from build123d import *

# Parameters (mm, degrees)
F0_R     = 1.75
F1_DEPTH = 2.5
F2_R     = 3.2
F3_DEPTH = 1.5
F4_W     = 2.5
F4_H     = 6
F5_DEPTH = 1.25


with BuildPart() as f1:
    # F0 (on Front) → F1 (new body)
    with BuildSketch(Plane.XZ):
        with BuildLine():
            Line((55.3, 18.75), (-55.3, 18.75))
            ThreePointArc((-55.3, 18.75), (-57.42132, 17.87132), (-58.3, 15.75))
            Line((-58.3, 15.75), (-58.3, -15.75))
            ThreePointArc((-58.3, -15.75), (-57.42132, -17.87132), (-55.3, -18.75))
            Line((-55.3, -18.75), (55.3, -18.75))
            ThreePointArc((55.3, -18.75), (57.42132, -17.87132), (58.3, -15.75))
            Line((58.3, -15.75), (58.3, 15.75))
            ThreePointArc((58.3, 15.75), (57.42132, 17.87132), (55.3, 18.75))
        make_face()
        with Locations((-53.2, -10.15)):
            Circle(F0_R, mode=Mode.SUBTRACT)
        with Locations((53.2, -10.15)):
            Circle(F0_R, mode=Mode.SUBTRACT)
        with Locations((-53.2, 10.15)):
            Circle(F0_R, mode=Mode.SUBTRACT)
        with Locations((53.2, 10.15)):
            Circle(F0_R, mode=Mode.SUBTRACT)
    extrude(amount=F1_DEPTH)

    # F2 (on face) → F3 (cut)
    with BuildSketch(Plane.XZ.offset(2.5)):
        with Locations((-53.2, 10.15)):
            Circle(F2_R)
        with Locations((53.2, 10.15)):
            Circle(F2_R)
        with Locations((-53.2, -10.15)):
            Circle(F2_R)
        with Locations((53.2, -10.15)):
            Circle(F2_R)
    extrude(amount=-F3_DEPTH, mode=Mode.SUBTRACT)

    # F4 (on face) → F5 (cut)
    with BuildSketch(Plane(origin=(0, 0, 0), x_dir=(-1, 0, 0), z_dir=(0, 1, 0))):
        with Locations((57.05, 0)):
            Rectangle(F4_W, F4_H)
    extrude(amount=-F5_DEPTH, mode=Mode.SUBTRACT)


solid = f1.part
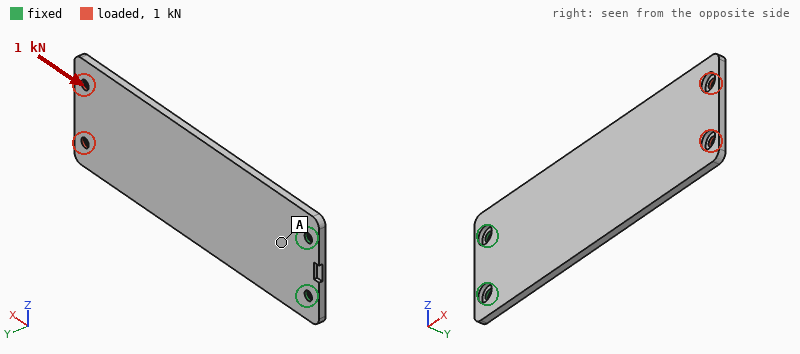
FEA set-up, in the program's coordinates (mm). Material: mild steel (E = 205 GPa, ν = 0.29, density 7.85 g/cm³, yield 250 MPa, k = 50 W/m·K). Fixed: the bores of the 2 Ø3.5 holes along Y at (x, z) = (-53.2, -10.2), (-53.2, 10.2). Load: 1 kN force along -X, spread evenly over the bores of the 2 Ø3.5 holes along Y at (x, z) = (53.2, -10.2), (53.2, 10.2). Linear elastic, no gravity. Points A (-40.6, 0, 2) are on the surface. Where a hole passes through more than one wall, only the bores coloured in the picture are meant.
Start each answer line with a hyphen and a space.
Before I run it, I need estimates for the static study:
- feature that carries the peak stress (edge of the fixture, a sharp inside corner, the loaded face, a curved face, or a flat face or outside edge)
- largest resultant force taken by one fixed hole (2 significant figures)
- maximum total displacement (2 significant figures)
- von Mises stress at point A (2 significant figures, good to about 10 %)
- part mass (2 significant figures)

- edge of the fixture
- 500 N
- 0.44 mm
- 28 MPa
- 84 g
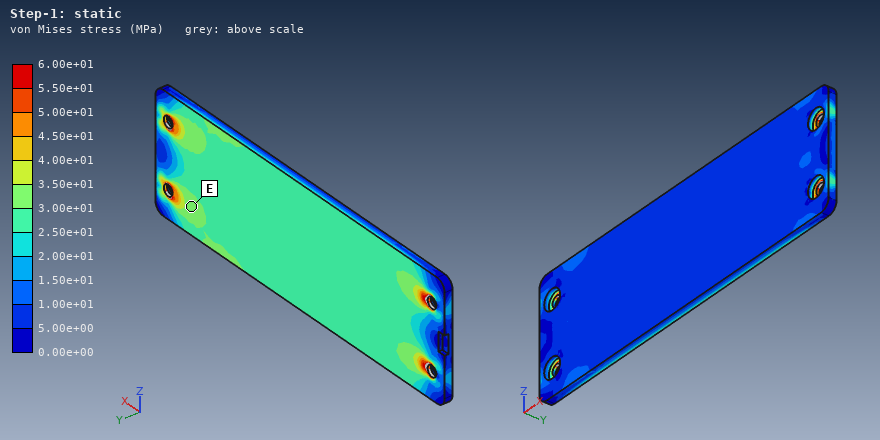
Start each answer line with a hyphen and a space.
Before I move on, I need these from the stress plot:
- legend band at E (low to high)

- 3.00e+01 to 3.50e+01 MPa
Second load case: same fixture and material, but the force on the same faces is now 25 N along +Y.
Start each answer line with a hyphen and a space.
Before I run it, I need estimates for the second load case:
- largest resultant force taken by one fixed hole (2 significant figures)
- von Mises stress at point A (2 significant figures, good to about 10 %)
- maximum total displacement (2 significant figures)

- 39 N
- 57 MPa
- 1.3 mm
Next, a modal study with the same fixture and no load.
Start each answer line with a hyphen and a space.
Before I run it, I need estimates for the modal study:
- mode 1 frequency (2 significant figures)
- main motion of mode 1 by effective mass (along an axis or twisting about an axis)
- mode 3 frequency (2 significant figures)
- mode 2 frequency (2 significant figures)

- 150 Hz
- along Y
- 980 Hz
- 960 Hz
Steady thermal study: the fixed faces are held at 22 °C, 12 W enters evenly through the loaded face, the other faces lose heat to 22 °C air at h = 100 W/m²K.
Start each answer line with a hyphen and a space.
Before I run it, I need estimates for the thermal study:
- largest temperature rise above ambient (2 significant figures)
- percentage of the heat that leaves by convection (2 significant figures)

- 67 K
- 98 %
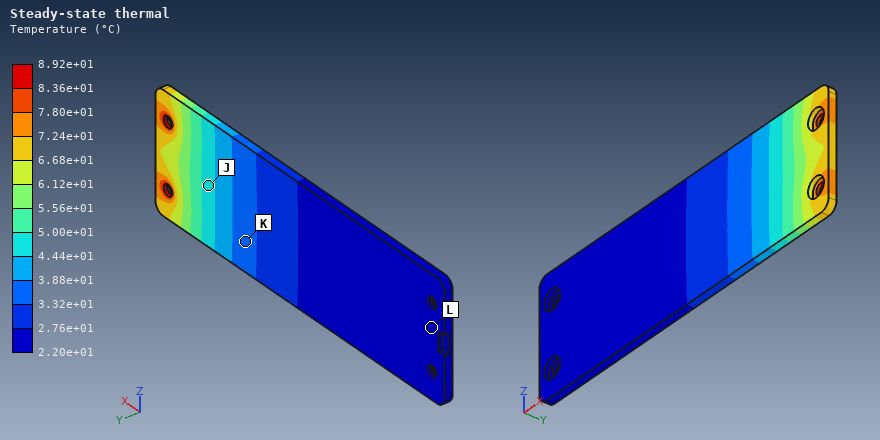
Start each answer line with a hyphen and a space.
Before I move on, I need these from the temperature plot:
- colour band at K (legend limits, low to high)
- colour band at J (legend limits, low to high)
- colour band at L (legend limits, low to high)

- 3.32e+01 to 3.88e+01 °C
- 4.44e+01 to 5.00e+01 °C
- 2.20e+01 to 2.76e+01 °C
